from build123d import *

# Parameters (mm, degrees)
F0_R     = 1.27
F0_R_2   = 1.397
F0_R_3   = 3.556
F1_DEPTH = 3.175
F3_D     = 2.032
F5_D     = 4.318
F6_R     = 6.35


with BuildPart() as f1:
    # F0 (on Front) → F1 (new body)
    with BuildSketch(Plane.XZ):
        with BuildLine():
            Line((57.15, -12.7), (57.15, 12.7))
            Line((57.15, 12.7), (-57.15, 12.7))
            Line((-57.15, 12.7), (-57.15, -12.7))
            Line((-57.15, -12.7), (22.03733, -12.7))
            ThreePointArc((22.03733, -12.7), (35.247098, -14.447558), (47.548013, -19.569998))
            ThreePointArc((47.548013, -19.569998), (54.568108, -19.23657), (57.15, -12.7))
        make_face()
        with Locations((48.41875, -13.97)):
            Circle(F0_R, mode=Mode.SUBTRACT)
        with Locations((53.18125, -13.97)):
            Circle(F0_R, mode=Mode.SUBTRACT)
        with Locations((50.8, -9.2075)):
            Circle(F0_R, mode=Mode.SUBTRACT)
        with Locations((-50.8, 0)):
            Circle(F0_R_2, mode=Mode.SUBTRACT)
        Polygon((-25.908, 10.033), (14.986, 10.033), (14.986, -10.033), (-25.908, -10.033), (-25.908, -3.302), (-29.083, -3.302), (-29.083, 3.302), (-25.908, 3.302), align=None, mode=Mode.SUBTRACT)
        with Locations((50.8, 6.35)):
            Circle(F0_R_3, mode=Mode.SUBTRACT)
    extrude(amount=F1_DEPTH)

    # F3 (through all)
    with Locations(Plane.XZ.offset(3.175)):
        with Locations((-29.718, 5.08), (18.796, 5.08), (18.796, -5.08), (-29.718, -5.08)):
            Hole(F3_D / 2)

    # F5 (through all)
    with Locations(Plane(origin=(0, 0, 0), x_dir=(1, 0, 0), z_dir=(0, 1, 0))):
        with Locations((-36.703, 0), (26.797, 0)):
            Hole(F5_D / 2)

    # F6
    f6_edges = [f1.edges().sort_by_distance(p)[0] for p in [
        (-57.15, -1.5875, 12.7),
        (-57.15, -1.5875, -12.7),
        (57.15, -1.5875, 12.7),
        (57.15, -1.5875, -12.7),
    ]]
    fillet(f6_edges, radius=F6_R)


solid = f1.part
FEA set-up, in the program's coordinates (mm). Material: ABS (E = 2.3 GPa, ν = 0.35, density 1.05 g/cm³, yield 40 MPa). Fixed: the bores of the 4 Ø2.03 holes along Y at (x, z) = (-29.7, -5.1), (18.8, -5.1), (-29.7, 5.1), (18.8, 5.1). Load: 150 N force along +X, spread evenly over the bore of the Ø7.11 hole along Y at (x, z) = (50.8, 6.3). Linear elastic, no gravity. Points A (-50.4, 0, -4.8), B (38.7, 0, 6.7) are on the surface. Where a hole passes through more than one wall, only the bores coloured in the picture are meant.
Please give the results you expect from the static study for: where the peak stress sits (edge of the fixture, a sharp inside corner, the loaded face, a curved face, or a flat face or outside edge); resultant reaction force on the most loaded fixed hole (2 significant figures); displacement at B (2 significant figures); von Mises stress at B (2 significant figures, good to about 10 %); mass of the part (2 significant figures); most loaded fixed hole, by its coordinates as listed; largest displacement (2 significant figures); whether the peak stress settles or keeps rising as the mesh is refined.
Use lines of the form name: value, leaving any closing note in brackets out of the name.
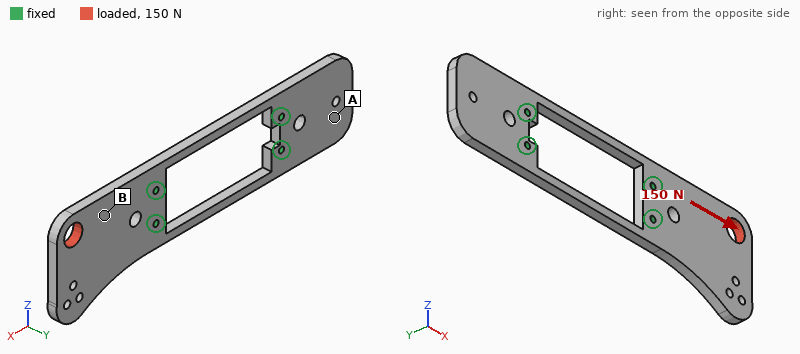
where the peak stress sits: edge of the fixture
resultant reaction force on the most loaded fixed hole: 140 N
displacement at B: 0.062 mm
von Mises stress at B: 3.1 MPa
mass of the part: 6.8 g
most loaded fixed hole, by its coordinates as listed: (18.8, 5.1)
largest displacement: 0.14 mm
whether the peak stress settles or keeps rising as the mesh is refined: keeps rising
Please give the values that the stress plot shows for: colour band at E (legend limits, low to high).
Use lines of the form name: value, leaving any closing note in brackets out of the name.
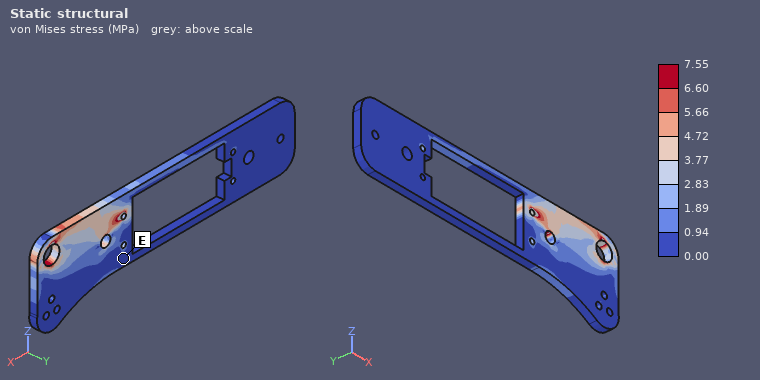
colour band at E: 0.00 to 0.94 MPa
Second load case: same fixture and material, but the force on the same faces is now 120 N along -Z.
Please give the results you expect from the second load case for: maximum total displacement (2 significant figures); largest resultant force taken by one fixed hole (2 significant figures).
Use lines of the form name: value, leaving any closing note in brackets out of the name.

maximum total displacement: 0.46 mm
largest resultant force taken by one fixed hole: 290 N
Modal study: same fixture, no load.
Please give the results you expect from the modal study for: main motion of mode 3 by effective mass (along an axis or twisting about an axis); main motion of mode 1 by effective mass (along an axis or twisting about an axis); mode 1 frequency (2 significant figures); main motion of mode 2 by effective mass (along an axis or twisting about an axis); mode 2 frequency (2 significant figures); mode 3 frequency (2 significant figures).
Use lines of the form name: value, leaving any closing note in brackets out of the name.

main motion of mode 3 by effective mass: twisting about X
main motion of mode 1 by effective mass: along Y
mode 1 frequency: 470 Hz
main motion of mode 2 by effective mass: along Y
mode 2 frequency: 960 Hz
mode 3 frequency: 1300 Hz
